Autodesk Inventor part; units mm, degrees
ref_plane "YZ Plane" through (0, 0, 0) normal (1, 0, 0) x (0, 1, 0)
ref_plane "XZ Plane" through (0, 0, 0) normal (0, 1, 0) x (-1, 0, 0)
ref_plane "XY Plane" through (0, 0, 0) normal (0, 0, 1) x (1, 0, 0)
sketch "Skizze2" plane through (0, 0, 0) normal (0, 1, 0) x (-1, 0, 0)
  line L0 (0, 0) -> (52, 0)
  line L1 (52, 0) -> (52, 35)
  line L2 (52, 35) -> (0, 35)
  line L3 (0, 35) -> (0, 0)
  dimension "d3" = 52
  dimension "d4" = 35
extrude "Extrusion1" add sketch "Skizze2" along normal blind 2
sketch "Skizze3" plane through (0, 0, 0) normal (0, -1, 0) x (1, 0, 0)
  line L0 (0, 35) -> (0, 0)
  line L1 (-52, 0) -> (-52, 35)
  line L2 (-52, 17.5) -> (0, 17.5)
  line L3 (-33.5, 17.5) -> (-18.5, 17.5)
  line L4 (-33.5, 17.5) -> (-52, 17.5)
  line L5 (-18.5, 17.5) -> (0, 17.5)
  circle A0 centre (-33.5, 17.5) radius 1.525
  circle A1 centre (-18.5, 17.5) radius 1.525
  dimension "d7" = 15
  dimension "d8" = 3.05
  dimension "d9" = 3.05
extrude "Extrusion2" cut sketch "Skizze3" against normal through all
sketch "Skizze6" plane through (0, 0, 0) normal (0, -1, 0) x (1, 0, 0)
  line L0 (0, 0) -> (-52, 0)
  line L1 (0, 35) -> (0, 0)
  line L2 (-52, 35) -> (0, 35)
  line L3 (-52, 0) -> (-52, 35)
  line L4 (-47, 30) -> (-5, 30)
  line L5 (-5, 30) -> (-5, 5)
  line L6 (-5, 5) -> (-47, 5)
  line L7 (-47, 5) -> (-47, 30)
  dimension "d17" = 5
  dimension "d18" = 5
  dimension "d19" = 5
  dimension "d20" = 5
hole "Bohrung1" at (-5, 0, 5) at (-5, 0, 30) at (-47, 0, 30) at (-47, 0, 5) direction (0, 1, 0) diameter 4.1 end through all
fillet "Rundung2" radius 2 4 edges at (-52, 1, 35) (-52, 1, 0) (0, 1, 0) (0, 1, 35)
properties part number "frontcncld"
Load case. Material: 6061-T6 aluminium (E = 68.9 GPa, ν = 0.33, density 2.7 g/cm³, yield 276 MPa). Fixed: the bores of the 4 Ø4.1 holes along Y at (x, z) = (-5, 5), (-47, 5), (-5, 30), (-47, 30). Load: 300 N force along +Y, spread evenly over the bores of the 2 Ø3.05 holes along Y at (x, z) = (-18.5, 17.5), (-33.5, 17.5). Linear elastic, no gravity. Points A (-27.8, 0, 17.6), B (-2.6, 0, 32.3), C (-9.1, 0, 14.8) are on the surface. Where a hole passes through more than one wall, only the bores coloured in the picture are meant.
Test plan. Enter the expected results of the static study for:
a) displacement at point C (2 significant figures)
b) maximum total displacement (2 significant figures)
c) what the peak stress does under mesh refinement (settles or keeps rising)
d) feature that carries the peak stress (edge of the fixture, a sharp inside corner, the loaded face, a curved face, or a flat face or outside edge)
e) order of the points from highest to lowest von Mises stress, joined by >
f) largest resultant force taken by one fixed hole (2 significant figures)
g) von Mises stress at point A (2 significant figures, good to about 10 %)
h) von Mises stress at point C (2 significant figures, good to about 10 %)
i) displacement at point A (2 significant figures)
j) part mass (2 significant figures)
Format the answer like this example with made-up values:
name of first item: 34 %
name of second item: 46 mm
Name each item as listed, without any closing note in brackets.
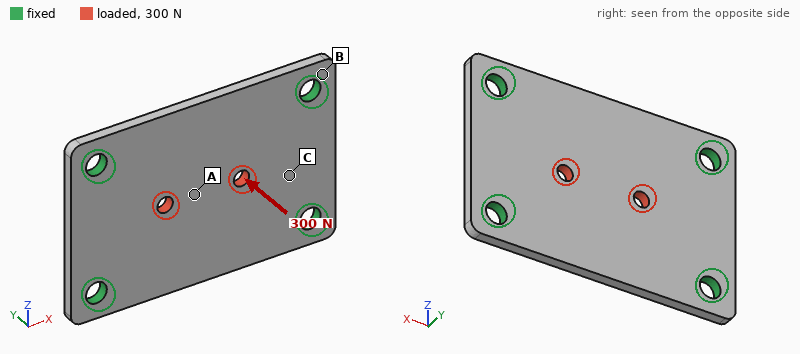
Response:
displacement at point C: 18 µm
maximum total displacement: 70 µm
what the peak stress does under mesh refinement: keeps rising
feature that carries the peak stress: edge of the fixture
order of the points from highest to lowest von Mises stress, joined by >: A > C > B
largest resultant force taken by one fixed hole: 75 N
von Mises stress at point A: 45 MPa
von Mises stress at point C: 28 MPa
displacement at point A: 70 µm
part mass: 9.4 g
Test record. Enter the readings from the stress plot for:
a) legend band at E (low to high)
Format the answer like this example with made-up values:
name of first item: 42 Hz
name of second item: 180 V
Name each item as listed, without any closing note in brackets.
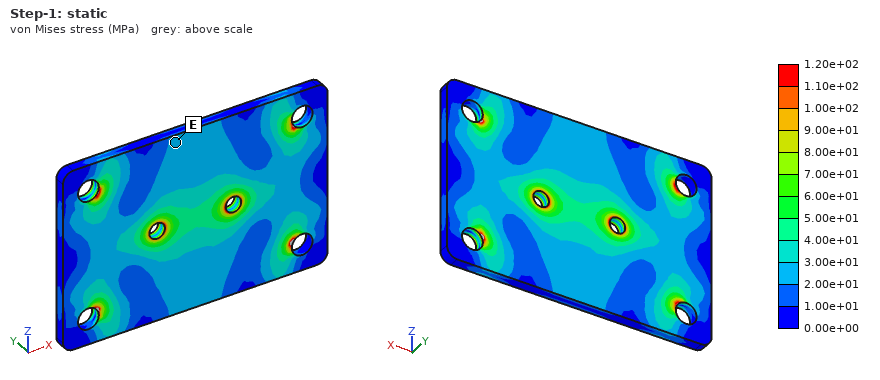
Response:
legend band at E: 2.00e+01 to 3.00e+01 MPa
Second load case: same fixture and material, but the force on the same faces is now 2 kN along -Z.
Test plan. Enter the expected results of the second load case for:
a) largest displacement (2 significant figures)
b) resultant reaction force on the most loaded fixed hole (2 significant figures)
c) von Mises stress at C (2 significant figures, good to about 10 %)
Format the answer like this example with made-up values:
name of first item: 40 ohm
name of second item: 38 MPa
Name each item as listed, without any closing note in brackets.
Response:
largest displacement: 13 µm
resultant reaction force on the most loaded fixed hole: 600 N
von Mises stress at C: 24 MPa
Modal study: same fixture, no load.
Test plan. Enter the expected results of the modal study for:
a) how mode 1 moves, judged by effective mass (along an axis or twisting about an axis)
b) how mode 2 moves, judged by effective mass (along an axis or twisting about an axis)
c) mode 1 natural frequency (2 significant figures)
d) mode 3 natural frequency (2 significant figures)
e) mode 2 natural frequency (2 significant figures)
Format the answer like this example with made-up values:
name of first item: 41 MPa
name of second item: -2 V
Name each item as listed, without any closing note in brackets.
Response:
how mode 1 moves, judged by effective mass: along Y
how mode 2 moves, judged by effective mass: twisting about X
mode 1 natural frequency: 6000 Hz
mode 3 natural frequency: 13 kHz
mode 2 natural frequency: 8100 Hz
